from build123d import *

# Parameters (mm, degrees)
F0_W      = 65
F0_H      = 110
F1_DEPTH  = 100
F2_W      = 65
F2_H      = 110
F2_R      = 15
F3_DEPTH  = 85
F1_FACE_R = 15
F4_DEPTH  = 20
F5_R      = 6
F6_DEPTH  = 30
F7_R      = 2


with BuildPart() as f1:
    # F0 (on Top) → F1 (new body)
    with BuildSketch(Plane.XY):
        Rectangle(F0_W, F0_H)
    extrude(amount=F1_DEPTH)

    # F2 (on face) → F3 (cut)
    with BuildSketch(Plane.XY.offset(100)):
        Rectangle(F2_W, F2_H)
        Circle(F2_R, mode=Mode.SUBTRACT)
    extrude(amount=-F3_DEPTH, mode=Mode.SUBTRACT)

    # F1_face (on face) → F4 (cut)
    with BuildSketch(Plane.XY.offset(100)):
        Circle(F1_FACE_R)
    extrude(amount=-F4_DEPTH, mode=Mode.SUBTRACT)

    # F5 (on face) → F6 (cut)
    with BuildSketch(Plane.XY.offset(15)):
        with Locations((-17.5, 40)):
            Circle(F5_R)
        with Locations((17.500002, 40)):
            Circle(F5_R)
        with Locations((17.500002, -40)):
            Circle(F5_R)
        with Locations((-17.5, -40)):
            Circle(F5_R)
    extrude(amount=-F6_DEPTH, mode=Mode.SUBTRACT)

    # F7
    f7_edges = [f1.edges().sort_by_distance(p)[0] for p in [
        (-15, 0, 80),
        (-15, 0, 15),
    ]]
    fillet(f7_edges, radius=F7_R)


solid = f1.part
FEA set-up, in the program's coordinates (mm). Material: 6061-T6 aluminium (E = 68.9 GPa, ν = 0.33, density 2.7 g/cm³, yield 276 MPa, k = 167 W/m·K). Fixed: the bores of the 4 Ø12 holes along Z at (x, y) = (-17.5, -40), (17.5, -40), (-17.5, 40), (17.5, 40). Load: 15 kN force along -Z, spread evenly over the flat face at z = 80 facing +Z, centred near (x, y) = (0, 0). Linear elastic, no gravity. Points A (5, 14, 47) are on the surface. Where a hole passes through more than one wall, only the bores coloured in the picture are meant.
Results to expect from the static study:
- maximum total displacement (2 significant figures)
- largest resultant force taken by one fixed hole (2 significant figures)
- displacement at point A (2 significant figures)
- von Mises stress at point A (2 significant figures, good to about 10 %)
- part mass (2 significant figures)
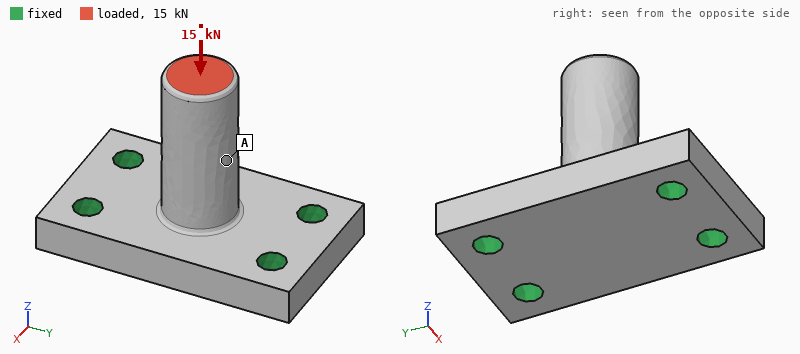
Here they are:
49 µm
3.8 kN
37 µm
21 MPa
400 g
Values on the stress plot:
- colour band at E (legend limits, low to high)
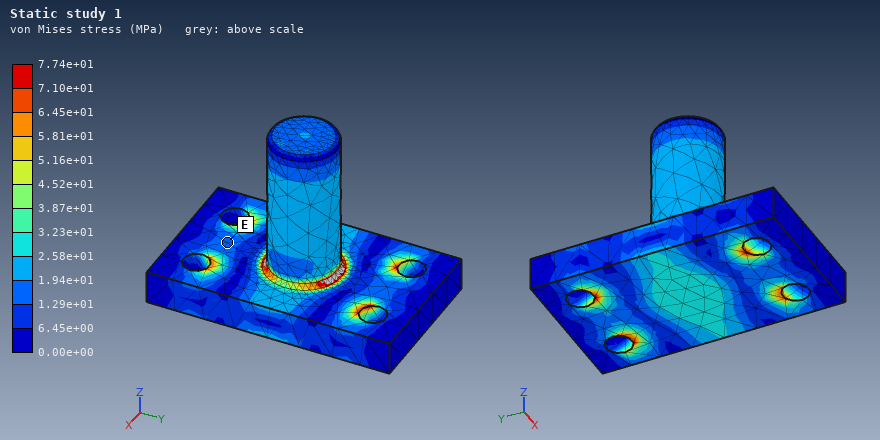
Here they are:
1.29e+01 to 1.94e+01 MPa
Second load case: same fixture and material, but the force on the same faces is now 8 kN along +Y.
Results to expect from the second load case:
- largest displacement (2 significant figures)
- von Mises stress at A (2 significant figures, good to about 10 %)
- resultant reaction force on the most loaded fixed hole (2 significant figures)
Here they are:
0.46 mm
95 MPa
5.6 kN
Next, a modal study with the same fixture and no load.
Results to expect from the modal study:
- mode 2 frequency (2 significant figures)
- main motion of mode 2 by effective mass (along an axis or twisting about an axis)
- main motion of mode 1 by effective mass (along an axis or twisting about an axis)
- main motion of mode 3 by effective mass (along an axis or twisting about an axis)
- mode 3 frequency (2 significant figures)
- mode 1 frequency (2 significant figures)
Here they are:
3500 Hz
along Y
along X
along Z
7700 Hz
3100 Hz
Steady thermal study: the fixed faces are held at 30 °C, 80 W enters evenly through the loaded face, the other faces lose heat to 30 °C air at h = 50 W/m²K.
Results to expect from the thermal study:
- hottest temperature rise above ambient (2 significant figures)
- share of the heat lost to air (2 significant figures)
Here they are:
51 K
14 %
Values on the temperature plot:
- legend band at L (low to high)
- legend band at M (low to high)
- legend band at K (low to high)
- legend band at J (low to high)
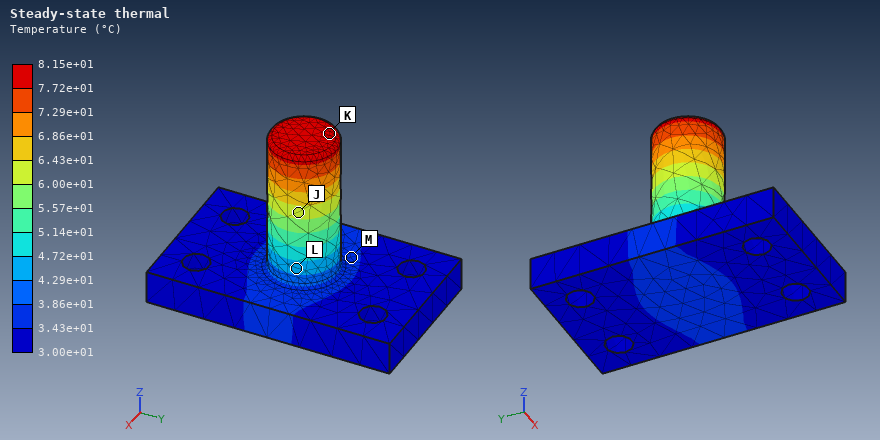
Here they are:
4.29e+01 to 4.72e+01 °C
3.43e+01 to 3.86e+01 °C
7.72e+01 to 8.15e+01 °C
6.00e+01 to 6.43e+01 °C
